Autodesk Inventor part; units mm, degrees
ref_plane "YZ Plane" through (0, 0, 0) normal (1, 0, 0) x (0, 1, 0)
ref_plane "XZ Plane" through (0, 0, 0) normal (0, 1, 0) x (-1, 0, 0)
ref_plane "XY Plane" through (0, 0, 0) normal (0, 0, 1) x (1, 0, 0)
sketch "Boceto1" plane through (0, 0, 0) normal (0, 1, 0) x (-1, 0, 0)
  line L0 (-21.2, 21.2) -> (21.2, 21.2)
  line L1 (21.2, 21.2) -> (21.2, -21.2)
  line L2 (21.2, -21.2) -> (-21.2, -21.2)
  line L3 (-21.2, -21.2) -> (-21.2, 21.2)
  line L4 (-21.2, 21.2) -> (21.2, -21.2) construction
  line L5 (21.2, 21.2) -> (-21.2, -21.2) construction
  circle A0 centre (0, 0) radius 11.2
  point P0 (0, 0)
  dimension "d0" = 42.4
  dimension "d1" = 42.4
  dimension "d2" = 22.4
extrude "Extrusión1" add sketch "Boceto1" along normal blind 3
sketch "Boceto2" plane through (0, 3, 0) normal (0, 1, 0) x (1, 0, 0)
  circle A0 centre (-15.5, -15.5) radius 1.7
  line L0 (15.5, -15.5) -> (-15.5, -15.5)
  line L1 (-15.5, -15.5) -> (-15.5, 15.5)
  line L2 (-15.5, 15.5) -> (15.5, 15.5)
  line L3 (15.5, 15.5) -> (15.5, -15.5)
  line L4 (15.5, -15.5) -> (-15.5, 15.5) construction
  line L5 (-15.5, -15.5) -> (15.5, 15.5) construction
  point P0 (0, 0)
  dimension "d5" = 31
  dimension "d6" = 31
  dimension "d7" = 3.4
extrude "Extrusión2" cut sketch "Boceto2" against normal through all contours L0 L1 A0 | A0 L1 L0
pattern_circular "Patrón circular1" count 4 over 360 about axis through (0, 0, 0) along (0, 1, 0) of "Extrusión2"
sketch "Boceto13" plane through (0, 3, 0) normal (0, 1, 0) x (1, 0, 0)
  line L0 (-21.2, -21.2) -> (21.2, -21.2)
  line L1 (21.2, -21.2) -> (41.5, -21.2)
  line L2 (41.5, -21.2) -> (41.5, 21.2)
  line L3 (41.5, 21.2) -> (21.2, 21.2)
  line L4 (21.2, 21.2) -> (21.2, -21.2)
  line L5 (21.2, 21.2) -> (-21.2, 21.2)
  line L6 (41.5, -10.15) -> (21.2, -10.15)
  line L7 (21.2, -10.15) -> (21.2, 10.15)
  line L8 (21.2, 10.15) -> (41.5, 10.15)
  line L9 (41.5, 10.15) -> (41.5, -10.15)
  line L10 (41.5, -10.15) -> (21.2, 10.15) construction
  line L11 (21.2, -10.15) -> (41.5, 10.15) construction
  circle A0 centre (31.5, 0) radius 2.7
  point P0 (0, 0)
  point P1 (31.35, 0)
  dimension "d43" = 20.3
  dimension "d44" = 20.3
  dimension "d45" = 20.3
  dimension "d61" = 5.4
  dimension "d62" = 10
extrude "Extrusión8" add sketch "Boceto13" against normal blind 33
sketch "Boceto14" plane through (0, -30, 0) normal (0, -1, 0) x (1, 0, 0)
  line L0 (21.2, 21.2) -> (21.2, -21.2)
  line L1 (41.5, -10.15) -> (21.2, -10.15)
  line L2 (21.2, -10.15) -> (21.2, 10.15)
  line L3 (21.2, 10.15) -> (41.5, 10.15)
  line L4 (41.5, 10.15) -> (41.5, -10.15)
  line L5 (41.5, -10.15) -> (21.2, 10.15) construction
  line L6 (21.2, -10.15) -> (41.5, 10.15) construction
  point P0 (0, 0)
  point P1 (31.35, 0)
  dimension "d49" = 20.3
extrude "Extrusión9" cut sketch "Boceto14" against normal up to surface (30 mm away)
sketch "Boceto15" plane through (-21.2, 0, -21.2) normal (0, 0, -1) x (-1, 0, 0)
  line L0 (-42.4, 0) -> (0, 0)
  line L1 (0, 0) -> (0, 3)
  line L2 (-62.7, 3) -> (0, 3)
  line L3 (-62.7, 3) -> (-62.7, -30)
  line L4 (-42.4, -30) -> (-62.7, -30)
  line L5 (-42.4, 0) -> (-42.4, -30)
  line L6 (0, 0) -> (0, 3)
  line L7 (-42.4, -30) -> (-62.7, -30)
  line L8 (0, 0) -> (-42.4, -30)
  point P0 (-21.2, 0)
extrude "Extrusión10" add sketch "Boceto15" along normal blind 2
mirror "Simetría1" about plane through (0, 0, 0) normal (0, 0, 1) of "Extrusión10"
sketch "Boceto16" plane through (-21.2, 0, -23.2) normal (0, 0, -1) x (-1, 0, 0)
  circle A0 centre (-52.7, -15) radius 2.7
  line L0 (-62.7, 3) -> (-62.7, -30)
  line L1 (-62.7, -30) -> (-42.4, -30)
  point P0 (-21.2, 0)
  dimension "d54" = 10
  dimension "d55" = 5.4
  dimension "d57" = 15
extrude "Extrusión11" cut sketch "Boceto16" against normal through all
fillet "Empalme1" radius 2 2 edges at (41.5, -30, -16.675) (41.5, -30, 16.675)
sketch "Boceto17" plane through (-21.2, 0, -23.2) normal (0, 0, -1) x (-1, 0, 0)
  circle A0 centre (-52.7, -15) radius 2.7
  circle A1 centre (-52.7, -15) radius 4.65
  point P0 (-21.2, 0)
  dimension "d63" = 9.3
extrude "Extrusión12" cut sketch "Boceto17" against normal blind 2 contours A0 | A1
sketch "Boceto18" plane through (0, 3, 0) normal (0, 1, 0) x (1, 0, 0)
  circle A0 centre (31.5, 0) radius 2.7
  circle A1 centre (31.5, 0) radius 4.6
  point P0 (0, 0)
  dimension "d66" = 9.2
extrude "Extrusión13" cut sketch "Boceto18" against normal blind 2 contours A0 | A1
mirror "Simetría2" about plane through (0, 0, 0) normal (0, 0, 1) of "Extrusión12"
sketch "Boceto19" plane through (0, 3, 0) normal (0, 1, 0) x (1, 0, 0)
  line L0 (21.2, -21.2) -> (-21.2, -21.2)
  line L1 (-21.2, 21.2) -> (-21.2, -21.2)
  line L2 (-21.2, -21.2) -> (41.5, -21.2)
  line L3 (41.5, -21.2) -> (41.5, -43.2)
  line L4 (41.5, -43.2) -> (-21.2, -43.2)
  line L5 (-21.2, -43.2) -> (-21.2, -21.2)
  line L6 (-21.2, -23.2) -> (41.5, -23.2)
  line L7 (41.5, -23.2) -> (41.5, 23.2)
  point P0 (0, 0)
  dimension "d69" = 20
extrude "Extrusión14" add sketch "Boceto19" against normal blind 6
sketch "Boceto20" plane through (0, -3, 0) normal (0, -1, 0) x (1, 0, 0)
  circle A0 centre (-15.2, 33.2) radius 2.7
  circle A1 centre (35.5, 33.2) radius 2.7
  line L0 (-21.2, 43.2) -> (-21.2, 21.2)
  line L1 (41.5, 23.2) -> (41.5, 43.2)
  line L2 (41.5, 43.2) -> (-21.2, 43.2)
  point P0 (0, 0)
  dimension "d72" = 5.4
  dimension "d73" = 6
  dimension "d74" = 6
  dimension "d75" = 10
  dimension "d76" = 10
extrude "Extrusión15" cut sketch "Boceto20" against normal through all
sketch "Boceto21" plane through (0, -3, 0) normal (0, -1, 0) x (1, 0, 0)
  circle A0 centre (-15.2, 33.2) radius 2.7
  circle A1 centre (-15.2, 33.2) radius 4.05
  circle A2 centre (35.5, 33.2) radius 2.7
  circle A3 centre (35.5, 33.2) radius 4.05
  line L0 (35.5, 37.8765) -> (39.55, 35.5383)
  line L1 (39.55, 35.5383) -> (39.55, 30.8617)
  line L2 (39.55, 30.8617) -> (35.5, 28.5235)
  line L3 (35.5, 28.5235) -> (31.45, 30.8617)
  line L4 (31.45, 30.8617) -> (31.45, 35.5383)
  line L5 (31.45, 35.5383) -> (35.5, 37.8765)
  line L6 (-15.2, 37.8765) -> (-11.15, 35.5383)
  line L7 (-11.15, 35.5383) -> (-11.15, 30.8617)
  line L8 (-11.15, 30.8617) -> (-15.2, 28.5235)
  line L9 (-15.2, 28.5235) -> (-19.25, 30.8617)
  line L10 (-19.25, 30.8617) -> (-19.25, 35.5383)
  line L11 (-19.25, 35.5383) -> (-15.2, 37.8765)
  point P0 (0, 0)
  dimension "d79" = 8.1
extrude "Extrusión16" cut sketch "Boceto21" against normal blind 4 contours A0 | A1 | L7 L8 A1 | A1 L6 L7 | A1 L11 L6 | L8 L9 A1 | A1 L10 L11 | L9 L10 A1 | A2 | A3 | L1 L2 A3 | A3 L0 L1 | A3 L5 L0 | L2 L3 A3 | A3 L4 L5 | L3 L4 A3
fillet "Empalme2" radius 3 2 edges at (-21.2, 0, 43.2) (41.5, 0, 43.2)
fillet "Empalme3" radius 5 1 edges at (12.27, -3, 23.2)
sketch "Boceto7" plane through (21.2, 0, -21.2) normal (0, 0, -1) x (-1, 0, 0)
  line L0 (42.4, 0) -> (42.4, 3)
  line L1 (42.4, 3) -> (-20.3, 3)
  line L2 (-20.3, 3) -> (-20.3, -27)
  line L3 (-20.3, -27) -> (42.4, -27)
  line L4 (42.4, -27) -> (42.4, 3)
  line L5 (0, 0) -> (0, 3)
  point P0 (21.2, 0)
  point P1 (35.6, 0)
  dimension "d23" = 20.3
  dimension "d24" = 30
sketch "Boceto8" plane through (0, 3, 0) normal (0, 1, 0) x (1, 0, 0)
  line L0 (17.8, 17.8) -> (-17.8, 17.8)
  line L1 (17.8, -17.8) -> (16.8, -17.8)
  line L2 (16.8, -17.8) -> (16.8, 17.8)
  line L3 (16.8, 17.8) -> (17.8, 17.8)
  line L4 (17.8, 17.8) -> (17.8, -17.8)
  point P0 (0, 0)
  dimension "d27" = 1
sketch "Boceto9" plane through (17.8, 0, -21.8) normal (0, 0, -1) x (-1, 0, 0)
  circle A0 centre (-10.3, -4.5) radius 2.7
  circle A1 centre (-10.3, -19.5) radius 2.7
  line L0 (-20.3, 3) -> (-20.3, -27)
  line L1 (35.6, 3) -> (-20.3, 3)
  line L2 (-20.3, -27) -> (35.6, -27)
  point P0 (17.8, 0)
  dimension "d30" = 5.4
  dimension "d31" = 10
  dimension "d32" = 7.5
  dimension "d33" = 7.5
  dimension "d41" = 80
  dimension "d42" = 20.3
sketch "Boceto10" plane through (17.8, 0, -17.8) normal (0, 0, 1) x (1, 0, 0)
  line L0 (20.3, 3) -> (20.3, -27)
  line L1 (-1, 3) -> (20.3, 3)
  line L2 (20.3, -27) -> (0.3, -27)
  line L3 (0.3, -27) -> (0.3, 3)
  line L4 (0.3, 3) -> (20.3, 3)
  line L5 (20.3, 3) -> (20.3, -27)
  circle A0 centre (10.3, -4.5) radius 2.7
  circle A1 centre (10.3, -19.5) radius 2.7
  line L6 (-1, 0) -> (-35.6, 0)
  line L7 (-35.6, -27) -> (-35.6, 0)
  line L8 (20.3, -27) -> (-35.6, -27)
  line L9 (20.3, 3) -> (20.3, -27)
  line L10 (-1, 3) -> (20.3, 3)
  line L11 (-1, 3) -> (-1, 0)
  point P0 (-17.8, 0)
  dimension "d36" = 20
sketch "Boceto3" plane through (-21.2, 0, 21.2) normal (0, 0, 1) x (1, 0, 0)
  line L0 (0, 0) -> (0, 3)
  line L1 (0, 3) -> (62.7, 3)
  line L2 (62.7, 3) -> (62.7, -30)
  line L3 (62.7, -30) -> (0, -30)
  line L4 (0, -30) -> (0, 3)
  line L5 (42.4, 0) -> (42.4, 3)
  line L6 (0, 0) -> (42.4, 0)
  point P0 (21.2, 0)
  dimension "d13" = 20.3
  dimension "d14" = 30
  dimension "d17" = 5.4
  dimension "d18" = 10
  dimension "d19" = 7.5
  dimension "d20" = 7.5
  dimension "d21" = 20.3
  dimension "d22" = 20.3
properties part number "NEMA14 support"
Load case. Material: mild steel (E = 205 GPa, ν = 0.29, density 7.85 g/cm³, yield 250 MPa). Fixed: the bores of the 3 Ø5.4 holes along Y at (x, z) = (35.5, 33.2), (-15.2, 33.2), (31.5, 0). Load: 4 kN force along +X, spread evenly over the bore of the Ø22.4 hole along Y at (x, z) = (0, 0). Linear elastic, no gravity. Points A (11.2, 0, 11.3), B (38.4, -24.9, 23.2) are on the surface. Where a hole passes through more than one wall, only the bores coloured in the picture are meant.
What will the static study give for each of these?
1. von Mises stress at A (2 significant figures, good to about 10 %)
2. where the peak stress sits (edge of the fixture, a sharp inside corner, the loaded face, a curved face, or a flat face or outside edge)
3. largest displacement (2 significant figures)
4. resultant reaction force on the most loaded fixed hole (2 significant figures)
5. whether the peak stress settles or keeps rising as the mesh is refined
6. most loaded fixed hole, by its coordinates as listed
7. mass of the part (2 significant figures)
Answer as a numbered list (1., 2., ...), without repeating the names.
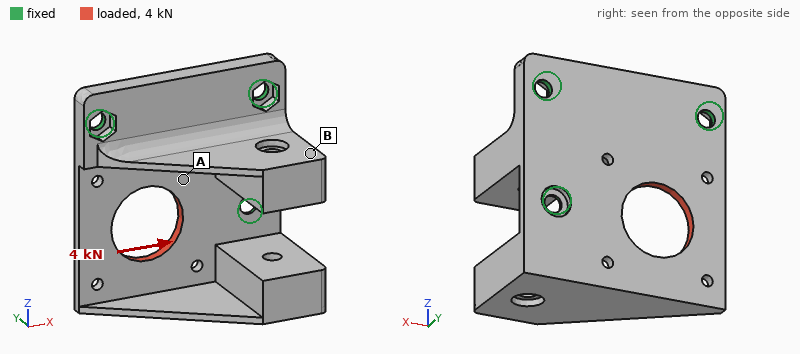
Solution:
1. 46 MPa
2. edge of the fixture
3. 43 µm
4. 2.4 kN
5. keeps rising
6. (31.5, 0)
7. 250 g
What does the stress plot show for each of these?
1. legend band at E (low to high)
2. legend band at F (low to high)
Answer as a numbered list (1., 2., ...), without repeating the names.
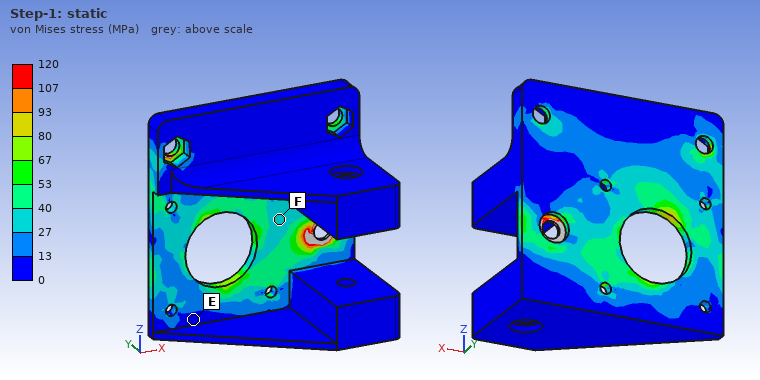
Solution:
1. 0 to 13 MPa
2. 27 to 40 MPa
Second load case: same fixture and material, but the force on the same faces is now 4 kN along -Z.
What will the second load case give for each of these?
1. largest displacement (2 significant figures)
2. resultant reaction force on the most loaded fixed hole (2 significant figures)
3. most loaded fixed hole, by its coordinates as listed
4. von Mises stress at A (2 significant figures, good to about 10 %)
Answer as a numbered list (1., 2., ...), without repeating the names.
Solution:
1. 14 µm
2. 2.4 kN
3. (-15.2, 33.2)
4. 26 MPa
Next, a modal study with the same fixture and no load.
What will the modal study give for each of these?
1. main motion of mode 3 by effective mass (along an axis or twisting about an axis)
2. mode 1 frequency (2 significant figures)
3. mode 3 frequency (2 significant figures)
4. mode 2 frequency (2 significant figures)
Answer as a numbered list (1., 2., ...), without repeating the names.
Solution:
1. along Y
2. 780 Hz
3. 4100 Hz
4. 1300 Hz
